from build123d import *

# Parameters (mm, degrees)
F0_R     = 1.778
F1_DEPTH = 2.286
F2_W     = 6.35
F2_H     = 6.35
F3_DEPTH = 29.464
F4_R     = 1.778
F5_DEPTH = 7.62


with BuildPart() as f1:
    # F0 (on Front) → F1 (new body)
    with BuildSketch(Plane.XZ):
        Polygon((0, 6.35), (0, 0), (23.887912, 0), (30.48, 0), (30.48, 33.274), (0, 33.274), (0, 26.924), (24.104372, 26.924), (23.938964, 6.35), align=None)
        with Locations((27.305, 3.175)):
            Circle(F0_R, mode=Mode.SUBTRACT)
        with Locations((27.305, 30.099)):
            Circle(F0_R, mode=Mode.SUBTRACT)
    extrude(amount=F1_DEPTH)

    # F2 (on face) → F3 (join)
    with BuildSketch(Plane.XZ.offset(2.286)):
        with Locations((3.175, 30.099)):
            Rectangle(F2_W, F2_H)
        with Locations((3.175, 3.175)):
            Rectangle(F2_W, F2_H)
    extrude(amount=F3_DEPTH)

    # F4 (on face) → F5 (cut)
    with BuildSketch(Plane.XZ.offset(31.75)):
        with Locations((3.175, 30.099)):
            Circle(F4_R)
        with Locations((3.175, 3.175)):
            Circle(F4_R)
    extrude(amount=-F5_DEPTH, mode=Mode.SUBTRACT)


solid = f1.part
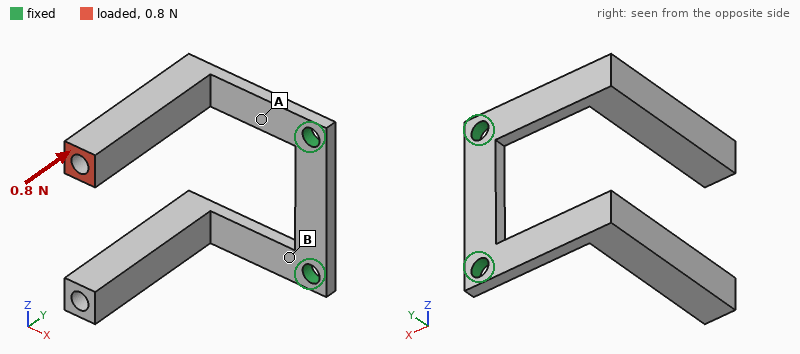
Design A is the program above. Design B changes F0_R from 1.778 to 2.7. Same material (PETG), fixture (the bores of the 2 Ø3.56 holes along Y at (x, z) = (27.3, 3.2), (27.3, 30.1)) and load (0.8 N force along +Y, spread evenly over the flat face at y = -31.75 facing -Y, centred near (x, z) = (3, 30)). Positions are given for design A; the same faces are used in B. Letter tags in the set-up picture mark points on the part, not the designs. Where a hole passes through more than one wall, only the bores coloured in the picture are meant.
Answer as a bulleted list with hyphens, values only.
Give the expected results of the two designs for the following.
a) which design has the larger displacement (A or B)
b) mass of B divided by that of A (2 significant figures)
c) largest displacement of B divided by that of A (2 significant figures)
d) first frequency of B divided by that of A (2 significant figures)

- A
- 0.98
- 0.91
- 1.0
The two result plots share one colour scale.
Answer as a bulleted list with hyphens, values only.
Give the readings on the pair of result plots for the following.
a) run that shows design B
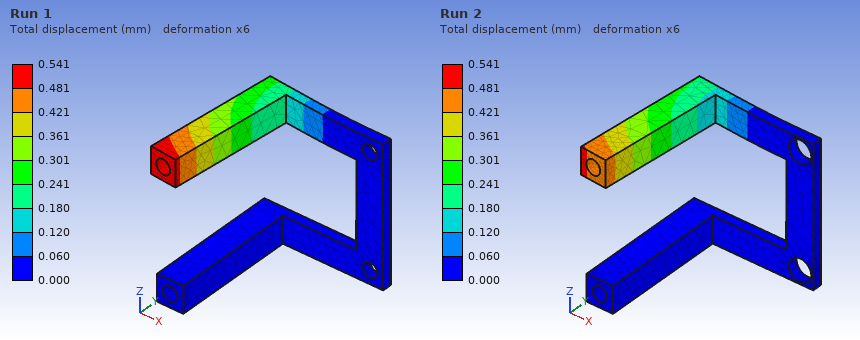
- Run 2
